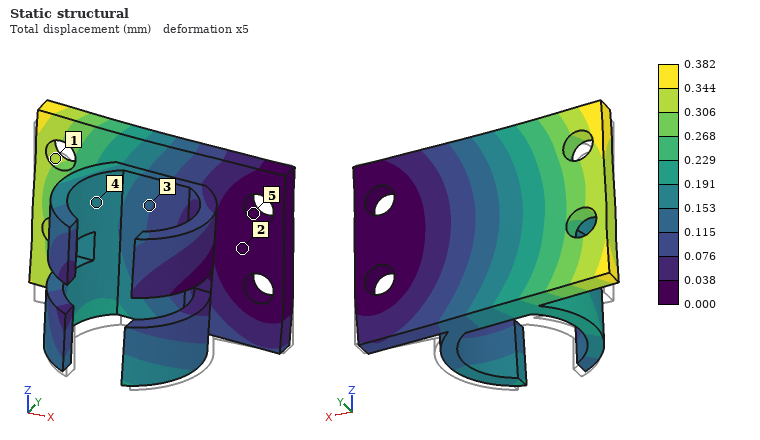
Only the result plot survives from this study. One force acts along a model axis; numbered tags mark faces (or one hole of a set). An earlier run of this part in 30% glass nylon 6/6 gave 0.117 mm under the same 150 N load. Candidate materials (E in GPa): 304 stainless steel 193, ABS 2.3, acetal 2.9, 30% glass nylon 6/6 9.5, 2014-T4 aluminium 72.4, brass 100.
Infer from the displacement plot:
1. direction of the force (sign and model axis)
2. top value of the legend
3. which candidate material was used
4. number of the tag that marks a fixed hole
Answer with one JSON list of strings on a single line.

["+Z", "0.382 mm", "acetal", "5"]
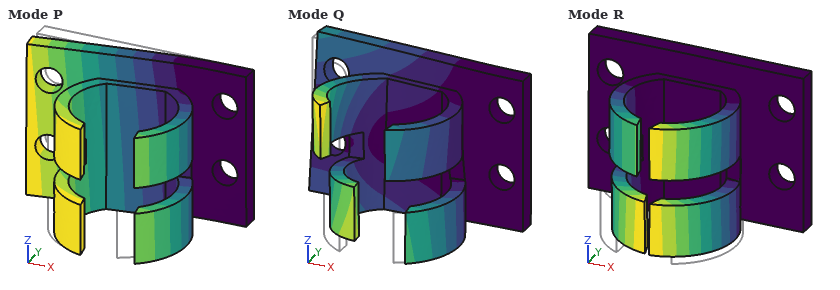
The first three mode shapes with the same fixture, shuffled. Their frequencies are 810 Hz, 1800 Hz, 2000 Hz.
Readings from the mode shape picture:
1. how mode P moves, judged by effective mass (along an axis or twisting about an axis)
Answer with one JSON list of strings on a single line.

["along Y"]
